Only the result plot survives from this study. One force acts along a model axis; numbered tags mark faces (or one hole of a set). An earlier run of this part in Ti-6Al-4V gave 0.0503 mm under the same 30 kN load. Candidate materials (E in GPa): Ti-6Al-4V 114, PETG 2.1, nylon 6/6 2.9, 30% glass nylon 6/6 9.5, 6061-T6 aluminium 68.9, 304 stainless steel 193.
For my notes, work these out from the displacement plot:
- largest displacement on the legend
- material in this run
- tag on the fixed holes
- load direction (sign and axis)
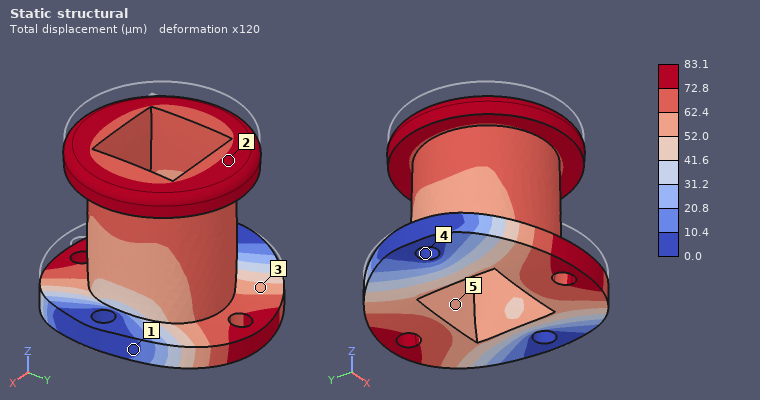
83.1 µm
6061-T6 aluminium
4
-Z
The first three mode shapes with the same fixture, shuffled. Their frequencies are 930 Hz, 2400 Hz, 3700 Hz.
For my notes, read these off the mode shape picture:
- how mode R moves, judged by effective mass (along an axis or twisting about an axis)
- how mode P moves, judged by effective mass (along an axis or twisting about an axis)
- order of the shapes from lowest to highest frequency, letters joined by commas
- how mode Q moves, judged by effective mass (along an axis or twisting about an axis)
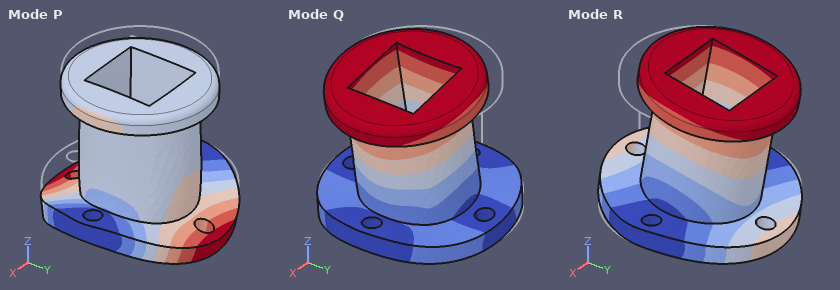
along Y
along Z
R, Q, P
along X
